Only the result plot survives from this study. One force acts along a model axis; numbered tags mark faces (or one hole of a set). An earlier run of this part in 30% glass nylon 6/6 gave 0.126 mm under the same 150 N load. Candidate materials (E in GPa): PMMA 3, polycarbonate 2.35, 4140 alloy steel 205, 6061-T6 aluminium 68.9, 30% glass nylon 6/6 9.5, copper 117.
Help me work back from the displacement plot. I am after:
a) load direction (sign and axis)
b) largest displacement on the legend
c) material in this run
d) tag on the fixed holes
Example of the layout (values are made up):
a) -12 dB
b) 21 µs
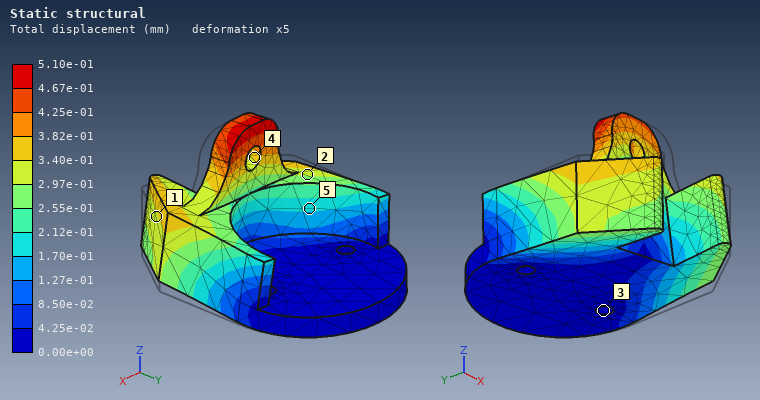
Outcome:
a) -X
b) 5.10e-01 mm
c) polycarbonate
d) 3
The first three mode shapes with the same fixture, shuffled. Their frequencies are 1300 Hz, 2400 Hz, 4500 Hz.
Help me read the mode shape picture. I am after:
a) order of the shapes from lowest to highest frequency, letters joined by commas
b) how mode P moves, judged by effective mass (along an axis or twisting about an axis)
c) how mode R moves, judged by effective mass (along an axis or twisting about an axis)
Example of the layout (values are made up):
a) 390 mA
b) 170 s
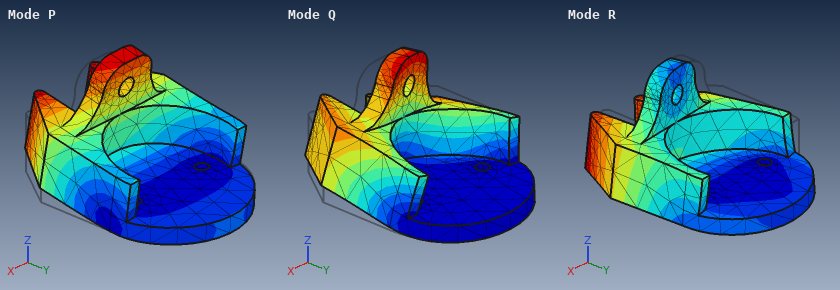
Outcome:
a) P, Q, R
b) along Z
c) along X
